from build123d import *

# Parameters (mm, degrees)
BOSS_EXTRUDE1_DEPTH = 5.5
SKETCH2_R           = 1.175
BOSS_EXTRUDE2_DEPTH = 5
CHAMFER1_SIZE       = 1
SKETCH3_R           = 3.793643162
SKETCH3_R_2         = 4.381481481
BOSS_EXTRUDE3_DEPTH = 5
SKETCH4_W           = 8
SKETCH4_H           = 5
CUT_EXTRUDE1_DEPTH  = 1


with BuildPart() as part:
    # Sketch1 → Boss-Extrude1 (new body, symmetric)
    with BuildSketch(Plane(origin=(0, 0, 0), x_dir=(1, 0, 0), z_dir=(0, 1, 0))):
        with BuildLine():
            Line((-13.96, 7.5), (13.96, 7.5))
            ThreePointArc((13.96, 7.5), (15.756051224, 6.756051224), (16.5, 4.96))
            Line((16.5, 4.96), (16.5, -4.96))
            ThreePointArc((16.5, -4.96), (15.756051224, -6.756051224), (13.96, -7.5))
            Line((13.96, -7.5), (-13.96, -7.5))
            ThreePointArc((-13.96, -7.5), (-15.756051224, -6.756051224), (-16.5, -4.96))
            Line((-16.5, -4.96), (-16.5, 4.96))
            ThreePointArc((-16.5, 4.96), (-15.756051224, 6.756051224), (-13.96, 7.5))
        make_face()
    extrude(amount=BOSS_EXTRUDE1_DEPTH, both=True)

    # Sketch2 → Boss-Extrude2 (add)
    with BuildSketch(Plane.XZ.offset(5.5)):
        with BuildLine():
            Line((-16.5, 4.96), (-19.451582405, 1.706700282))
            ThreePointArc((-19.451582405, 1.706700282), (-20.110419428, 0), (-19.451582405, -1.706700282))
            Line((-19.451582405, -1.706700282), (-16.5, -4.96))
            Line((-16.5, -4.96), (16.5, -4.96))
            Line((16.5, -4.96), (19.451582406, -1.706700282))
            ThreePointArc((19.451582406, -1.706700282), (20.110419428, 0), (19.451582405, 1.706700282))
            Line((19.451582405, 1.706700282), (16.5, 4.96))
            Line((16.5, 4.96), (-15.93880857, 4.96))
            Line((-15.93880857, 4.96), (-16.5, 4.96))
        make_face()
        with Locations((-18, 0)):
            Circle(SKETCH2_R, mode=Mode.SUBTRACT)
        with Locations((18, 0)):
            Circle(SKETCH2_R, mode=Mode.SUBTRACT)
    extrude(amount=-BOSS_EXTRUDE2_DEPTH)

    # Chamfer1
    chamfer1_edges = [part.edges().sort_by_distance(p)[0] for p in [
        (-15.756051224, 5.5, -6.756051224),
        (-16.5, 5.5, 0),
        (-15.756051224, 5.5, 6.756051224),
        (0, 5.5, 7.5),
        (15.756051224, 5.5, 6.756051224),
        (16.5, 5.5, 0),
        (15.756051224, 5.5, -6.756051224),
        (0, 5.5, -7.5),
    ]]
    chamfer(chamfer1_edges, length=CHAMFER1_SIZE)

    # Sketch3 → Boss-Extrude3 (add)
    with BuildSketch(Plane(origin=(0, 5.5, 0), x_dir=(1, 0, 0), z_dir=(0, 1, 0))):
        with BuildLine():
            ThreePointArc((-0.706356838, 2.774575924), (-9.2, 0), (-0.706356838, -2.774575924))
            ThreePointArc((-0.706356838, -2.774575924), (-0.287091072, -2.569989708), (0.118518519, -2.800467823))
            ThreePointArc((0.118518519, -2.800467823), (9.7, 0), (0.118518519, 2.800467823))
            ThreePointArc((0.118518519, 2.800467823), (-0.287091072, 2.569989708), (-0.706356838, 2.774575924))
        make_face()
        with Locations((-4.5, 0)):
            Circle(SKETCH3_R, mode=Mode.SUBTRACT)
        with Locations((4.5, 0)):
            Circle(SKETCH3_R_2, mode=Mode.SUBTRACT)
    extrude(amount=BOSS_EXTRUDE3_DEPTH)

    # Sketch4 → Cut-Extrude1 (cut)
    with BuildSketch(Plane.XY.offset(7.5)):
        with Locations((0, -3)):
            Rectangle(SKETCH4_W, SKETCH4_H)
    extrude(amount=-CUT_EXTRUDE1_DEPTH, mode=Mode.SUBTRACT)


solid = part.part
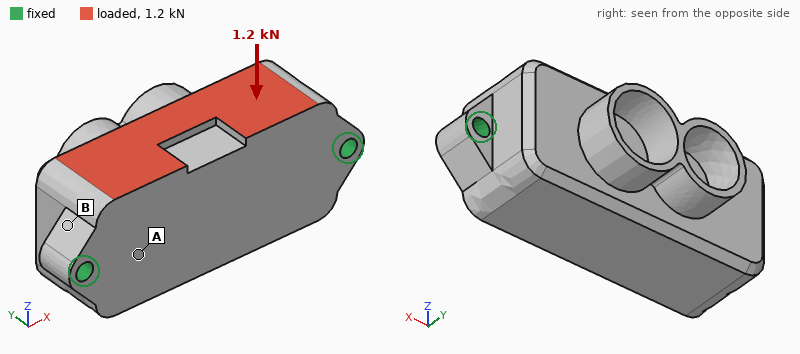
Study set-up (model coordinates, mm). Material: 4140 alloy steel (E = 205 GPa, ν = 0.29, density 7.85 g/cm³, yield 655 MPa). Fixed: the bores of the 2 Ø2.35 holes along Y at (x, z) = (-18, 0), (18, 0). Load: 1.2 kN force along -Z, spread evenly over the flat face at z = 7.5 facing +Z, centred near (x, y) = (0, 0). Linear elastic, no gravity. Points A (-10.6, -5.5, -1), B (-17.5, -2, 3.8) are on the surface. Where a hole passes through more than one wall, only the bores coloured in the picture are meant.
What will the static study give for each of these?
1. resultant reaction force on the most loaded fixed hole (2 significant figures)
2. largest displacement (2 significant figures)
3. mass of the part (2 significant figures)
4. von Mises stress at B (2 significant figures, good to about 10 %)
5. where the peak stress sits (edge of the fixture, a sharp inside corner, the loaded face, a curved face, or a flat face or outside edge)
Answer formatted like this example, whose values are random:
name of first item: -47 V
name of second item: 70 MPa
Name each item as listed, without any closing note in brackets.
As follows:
resultant reaction force on the most loaded fixed hole: 600 N
largest displacement: 6.2 µm
mass of the part: 45 g
von Mises stress at B: 36 MPa
where the peak stress sits: edge of the fixture
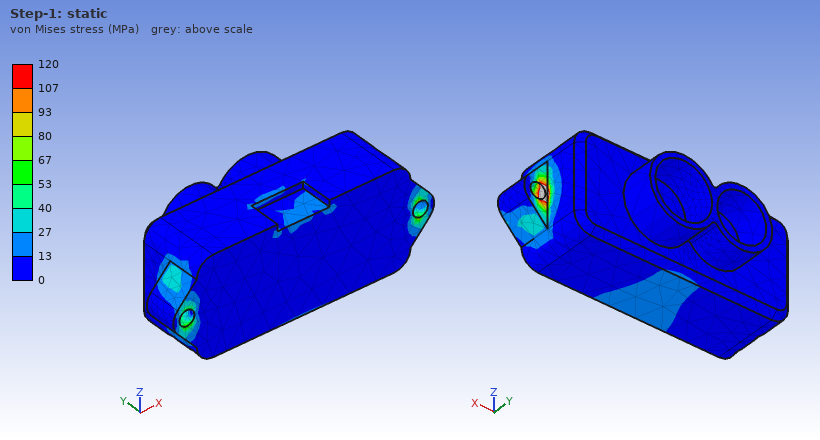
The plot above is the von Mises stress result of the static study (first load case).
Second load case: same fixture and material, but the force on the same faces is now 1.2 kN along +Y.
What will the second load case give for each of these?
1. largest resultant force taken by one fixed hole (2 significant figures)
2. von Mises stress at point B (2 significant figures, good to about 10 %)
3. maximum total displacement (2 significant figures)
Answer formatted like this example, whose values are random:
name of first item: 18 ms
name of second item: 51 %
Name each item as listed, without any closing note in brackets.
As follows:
largest resultant force taken by one fixed hole: 710 N
von Mises stress at point B: 100 MPa
maximum total displacement: 14 µm
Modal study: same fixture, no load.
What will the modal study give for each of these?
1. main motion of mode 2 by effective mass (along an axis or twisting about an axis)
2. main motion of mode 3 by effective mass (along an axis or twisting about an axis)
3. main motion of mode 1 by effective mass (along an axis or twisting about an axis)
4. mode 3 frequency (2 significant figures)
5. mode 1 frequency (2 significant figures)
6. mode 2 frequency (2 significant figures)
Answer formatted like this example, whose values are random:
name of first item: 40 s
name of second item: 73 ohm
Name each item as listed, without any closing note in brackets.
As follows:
main motion of mode 2 by effective mass: along Y
main motion of mode 3 by effective mass: along Z
main motion of mode 1 by effective mass: along Z
mode 3 frequency: 24 kHz
mode 1 frequency: 12 kHz
mode 2 frequency: 20 kHz
